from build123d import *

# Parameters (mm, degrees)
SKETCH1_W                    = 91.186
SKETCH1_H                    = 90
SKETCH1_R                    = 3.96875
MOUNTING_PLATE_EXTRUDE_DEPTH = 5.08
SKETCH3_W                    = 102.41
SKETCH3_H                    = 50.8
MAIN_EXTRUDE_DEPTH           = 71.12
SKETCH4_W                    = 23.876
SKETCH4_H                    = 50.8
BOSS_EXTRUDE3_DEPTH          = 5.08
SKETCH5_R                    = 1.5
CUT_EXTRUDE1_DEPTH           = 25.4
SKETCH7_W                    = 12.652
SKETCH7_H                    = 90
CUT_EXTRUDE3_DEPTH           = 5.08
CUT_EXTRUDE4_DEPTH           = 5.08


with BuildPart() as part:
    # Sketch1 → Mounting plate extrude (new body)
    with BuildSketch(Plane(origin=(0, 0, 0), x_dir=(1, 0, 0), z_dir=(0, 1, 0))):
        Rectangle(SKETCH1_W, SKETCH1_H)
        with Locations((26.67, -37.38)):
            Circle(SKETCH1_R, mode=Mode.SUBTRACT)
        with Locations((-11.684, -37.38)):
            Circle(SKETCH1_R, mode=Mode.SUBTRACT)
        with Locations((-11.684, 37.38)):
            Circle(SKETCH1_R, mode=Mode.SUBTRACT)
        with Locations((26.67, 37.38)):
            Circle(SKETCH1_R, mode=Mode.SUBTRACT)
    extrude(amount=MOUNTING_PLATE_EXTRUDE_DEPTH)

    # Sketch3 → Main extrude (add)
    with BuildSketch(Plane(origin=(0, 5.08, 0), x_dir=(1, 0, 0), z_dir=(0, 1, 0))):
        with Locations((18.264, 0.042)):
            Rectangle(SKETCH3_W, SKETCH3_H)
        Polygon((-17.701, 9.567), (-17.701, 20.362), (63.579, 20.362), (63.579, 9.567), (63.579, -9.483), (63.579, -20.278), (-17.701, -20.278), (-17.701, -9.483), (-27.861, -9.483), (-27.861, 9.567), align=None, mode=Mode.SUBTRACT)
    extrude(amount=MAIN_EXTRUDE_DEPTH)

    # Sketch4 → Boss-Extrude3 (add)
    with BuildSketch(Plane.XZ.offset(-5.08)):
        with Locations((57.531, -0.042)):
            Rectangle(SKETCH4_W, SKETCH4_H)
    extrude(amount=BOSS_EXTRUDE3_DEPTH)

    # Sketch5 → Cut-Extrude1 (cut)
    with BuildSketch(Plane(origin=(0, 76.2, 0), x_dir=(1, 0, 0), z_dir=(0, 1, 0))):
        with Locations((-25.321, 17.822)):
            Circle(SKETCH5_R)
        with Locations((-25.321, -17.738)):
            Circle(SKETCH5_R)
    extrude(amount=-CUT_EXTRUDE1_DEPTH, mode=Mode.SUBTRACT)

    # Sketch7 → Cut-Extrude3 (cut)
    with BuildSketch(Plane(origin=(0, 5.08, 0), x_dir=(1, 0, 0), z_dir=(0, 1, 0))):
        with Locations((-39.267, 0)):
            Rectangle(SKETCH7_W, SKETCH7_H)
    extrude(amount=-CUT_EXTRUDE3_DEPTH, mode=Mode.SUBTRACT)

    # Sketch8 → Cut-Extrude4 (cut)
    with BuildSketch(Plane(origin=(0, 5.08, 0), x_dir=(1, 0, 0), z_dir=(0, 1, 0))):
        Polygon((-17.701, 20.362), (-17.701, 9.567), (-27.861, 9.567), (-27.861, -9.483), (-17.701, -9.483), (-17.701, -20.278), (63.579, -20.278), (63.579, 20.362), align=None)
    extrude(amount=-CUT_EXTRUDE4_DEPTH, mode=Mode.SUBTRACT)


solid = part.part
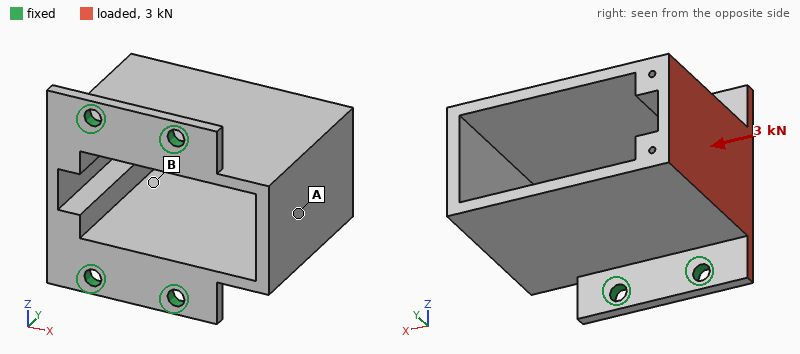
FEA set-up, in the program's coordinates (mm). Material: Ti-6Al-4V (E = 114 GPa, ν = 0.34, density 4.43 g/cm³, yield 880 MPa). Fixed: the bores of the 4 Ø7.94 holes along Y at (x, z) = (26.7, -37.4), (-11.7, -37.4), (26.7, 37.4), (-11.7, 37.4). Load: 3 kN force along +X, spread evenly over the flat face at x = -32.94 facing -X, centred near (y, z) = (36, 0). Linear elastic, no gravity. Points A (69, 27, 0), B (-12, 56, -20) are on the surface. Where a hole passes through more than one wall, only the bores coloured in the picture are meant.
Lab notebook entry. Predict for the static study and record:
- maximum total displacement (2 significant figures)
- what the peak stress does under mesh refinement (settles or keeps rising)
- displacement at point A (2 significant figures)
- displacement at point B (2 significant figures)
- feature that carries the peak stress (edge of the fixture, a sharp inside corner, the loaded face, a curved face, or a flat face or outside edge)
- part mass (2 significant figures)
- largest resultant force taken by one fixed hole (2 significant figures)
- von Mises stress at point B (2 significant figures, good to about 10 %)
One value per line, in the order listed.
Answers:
67 µm
keeps rising
43 µm
41 µm
edge of the fixture
640 g
1.4 kN
12 MPa
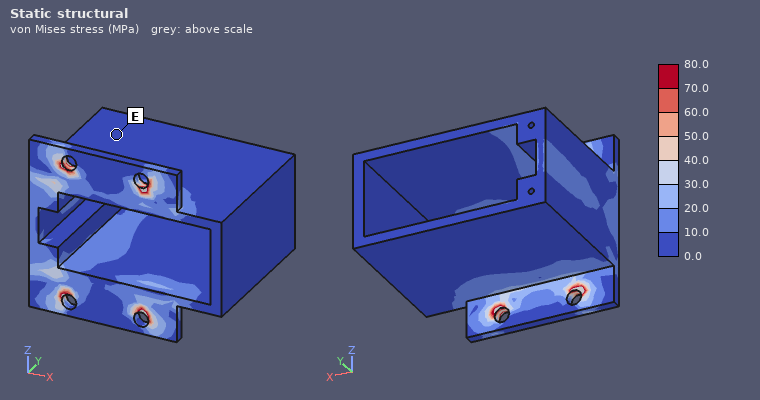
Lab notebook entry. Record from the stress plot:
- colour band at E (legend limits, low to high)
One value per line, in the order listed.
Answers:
0.0 to 10.0 MPa
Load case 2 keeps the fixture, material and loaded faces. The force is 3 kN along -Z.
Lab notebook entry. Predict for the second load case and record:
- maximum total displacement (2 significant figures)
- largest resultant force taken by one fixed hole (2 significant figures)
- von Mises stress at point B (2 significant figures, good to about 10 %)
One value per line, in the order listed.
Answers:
46 µm
2.1 kN
8.7 MPa
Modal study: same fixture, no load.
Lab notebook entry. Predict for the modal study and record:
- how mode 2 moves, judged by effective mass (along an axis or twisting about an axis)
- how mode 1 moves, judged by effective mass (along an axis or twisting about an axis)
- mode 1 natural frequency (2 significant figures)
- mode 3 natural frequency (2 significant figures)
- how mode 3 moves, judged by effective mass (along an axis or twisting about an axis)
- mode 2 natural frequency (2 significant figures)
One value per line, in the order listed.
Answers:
along Z
along X
1500 Hz
2500 Hz
along Z
1800 Hz
